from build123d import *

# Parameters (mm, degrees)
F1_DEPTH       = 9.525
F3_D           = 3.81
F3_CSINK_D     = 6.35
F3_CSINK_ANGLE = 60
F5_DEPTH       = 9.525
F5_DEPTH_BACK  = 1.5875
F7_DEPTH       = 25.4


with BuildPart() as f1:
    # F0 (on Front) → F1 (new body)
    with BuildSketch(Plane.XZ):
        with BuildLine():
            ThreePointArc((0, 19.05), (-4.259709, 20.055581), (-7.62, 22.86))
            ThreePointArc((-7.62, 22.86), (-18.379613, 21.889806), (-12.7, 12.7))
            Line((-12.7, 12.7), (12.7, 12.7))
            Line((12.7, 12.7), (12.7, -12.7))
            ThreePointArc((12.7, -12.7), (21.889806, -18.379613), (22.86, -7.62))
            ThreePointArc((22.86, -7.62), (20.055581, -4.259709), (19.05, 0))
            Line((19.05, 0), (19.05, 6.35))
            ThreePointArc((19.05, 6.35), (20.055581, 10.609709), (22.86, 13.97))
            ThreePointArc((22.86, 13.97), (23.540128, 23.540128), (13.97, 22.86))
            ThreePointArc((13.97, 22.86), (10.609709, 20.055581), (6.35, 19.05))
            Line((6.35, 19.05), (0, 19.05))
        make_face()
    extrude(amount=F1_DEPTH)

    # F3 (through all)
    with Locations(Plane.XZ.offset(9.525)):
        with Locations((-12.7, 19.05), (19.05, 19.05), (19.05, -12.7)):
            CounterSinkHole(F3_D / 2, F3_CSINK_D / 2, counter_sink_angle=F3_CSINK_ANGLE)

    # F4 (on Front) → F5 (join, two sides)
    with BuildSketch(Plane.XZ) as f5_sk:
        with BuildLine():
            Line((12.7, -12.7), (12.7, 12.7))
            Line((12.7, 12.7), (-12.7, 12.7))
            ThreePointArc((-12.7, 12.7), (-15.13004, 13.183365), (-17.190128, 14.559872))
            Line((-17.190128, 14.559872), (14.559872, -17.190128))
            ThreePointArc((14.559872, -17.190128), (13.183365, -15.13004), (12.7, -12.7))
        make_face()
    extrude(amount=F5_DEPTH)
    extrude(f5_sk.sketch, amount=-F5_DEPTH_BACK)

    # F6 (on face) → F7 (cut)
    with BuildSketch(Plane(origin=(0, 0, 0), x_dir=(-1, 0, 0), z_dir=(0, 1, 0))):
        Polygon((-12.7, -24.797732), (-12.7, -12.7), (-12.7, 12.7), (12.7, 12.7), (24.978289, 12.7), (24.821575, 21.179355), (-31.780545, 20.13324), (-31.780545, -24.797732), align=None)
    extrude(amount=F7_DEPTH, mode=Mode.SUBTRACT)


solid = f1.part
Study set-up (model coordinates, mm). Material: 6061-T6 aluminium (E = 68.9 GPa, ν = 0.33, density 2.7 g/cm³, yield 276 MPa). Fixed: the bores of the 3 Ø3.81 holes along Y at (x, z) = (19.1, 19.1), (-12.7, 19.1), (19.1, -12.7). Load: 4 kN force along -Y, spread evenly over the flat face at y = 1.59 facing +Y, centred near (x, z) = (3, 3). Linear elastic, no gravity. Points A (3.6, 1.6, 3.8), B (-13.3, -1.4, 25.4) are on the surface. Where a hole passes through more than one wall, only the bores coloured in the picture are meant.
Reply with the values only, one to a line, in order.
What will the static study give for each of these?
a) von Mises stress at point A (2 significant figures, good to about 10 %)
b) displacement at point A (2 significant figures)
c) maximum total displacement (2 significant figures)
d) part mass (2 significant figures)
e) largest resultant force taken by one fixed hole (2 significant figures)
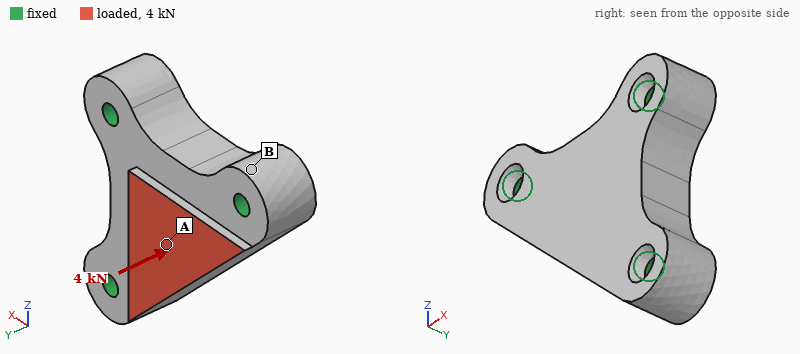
34 MPa
23 µm
31 µm
28 g
1.6 kN
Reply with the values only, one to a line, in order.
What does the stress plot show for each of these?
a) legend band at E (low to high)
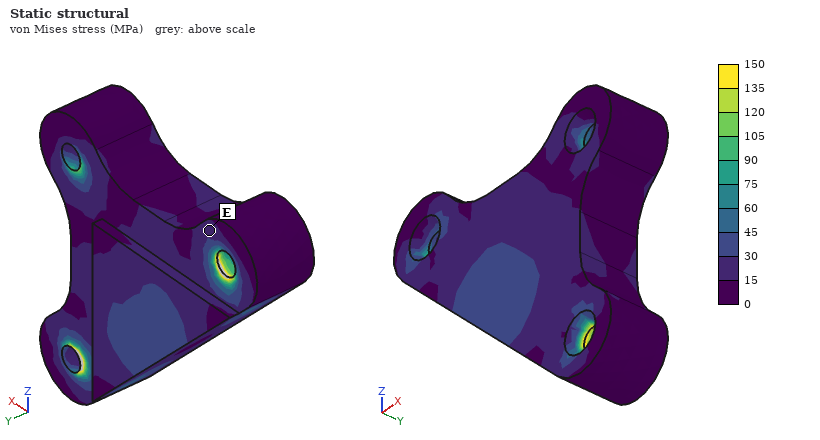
15 to 30 MPa
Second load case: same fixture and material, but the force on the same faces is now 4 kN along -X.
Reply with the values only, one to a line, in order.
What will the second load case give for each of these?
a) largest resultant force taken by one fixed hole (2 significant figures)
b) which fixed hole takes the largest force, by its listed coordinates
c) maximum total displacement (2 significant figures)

2.0 kN
(19.1, 19.1)
16 µm
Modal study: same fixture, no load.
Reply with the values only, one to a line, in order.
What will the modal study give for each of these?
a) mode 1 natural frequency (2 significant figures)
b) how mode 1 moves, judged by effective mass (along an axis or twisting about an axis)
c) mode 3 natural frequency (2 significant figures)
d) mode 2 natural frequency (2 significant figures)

19 kHz
along Y
37 kHz
33 kHz
